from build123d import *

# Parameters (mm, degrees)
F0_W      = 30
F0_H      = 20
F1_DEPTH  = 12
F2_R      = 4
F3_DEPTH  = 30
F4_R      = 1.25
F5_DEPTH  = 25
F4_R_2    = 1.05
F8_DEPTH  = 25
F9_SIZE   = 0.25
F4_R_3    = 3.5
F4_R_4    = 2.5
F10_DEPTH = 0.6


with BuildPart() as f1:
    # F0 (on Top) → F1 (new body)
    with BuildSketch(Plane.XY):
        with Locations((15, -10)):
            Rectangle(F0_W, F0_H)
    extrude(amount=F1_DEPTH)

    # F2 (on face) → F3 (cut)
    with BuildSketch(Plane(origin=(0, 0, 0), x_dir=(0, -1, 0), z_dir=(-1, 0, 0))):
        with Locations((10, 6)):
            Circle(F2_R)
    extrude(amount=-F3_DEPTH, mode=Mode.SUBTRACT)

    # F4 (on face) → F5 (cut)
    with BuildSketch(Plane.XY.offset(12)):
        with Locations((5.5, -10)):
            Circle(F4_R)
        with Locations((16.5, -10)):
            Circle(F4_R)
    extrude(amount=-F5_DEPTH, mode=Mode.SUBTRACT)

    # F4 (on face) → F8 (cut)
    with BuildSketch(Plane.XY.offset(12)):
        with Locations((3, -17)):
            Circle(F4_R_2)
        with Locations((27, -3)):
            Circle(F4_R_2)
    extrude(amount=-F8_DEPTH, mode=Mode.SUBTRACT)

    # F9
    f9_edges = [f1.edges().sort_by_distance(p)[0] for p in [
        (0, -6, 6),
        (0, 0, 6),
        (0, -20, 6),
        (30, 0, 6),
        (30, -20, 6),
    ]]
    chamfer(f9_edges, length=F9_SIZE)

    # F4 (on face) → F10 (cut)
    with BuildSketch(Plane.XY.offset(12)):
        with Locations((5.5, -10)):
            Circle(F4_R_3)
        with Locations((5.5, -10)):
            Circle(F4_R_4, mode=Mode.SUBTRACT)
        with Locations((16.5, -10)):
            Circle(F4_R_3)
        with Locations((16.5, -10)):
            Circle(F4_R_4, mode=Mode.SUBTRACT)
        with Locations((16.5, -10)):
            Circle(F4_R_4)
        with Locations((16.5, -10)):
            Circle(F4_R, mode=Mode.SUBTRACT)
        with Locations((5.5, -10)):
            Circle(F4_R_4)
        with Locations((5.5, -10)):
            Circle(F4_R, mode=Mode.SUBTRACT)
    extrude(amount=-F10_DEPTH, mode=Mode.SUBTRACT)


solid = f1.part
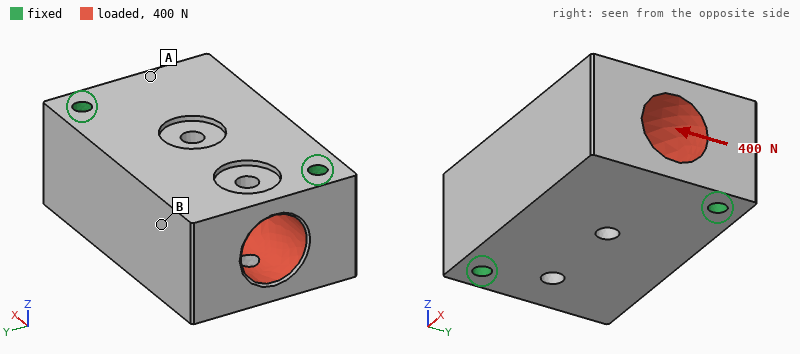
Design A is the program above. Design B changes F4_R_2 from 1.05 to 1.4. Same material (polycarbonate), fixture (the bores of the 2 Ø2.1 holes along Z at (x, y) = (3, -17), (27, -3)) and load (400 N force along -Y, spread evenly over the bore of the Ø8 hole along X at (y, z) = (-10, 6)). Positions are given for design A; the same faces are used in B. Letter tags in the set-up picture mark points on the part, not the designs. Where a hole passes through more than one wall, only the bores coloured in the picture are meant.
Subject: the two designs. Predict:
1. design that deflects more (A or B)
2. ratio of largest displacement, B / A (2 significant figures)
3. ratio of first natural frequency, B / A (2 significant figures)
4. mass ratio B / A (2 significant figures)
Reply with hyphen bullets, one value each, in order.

- A
- 0.92
- 1.0
- 0.99
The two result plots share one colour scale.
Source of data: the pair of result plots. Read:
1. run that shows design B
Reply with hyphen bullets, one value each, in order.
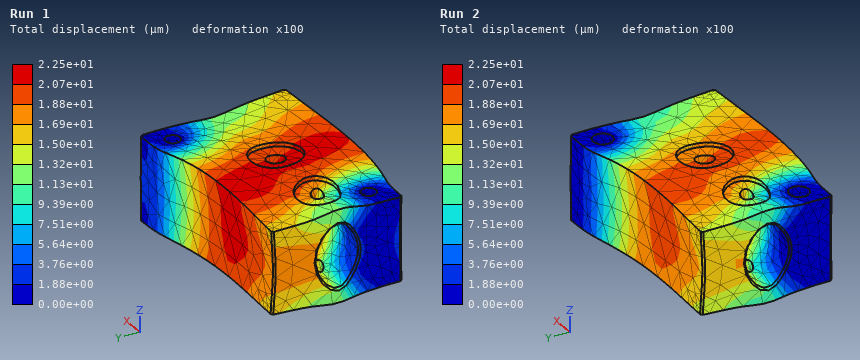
- Run 2
